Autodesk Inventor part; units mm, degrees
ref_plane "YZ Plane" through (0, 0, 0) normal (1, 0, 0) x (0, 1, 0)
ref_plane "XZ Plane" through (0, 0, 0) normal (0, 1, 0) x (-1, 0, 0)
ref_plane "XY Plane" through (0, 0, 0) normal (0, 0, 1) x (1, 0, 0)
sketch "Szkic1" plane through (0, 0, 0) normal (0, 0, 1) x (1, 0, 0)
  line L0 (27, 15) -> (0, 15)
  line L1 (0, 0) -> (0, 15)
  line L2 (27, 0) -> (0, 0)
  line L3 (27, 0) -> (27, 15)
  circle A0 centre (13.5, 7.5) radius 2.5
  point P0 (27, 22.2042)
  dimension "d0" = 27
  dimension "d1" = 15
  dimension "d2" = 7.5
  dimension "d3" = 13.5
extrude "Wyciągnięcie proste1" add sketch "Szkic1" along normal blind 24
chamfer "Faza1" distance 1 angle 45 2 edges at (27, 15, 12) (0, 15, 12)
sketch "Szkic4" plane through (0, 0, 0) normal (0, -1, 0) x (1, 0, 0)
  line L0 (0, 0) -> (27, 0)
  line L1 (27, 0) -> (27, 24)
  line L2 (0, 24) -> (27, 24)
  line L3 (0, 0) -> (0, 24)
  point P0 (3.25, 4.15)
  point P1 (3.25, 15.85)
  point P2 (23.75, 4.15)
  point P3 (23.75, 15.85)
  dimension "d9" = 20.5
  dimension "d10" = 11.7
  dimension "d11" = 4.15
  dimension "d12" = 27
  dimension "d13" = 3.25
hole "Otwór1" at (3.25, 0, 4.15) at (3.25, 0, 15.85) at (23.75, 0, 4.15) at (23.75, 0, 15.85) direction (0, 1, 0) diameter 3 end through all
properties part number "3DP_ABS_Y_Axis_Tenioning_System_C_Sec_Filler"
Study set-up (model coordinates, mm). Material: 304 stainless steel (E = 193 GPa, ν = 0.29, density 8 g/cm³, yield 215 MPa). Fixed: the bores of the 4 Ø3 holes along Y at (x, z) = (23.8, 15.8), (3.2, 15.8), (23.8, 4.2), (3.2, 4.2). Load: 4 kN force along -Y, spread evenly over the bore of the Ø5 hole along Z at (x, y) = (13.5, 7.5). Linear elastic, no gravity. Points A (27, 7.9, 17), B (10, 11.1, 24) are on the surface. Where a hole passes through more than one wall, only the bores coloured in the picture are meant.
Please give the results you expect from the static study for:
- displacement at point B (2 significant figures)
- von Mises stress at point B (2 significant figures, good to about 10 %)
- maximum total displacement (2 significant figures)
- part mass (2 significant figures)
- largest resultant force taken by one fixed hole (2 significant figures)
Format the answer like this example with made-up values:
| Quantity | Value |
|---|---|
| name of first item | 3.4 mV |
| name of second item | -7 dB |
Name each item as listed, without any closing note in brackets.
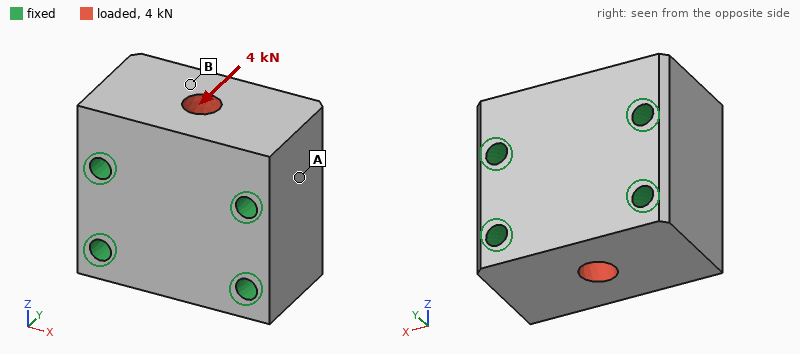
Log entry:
| Quantity | Value |
|---|---|
| displacement at point B | 0.94 µm |
| von Mises stress at point B | 11 MPa |
| maximum total displacement | 1.2 µm |
| part mass | 70 g |
| largest resultant force taken by one fixed hole | 1.2 kN |
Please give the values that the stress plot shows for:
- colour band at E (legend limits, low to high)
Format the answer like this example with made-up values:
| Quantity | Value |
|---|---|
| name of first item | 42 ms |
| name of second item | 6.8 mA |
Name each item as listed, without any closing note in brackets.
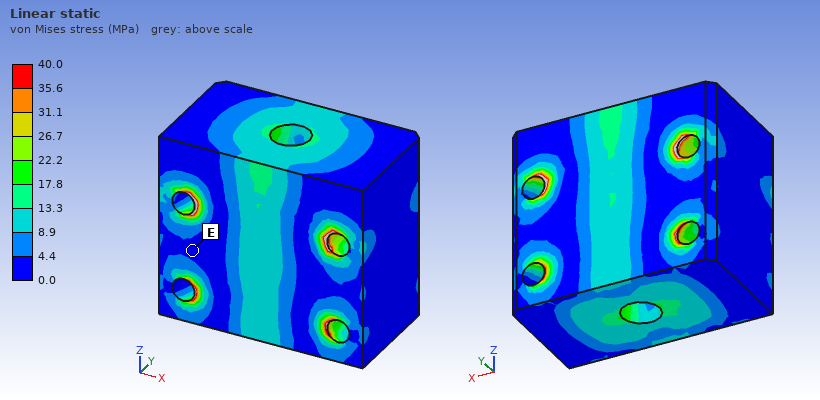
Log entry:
| Quantity | Value |
|---|---|
| colour band at E | 0.0 to 4.4 MPa |
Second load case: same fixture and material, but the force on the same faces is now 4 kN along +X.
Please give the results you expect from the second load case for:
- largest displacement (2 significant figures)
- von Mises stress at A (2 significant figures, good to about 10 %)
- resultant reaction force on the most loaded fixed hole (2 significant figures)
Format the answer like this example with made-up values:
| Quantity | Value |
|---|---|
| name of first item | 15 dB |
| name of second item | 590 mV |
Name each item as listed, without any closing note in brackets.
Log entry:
| Quantity | Value |
|---|---|
| largest displacement | 0.57 µm |
| von Mises stress at A | 5.6 MPa |
| resultant reaction force on the most loaded fixed hole | 1.2 kN |
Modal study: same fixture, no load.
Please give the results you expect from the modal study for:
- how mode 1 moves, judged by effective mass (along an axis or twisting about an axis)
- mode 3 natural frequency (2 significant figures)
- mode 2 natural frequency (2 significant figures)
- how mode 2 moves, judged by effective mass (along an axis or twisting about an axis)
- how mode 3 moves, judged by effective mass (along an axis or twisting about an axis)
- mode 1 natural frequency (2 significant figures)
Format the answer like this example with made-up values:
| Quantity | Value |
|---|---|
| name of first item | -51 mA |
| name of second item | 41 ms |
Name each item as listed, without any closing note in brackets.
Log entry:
| Quantity | Value |
|---|---|
| how mode 1 moves, judged by effective mass | along Y |
| mode 3 natural frequency | 71 kHz |
| mode 2 natural frequency | 67 kHz |
| how mode 2 moves, judged by effective mass | along Z |
| how mode 3 moves, judged by effective mass | along Y |
| mode 1 natural frequency | 58 kHz |
